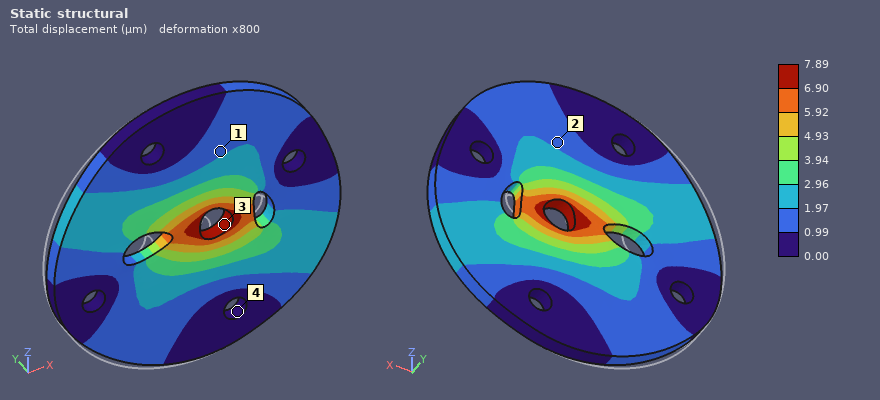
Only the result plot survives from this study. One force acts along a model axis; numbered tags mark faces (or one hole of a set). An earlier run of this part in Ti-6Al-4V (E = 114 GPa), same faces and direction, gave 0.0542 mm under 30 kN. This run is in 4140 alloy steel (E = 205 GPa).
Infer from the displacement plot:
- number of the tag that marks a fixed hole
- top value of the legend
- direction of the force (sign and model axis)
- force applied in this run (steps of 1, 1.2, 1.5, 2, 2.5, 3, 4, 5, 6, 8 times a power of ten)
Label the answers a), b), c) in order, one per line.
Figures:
a) 4
b) 7.89 µm
c) +X
d) 8 kN
